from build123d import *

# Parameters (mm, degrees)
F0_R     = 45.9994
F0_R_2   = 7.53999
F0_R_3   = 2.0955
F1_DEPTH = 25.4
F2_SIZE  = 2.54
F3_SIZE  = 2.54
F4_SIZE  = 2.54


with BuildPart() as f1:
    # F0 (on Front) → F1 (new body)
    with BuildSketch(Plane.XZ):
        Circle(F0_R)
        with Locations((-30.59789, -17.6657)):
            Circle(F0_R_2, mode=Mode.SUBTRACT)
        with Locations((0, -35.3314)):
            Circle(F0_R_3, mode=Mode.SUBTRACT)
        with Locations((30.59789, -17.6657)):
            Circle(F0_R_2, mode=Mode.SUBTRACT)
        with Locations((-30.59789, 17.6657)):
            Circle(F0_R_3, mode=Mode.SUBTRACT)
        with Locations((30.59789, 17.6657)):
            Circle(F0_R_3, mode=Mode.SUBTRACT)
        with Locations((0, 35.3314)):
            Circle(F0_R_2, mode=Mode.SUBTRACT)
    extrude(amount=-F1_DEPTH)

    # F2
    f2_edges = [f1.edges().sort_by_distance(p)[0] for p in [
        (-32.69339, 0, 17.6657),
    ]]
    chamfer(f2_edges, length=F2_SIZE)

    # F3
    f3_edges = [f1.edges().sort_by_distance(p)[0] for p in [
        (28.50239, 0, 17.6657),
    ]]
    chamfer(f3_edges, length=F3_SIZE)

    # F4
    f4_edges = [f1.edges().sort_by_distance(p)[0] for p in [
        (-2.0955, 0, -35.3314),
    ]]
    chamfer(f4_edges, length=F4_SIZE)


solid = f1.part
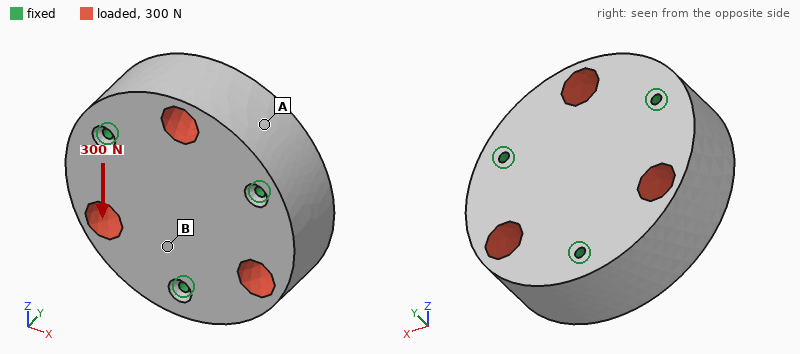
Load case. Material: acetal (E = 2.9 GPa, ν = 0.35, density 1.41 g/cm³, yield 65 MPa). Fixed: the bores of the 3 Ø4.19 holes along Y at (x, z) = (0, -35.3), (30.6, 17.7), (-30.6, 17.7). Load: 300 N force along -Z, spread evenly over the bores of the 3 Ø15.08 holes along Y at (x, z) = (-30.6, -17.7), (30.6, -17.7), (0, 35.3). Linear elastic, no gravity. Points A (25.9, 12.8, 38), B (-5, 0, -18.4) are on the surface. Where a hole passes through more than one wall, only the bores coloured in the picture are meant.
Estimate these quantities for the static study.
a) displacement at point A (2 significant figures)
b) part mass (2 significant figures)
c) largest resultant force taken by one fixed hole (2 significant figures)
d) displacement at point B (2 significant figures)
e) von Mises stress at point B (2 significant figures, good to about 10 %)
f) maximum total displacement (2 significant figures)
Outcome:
0.88 µm
220 g
110 N
0.91 µm
0.11 MPa
3.4 µm
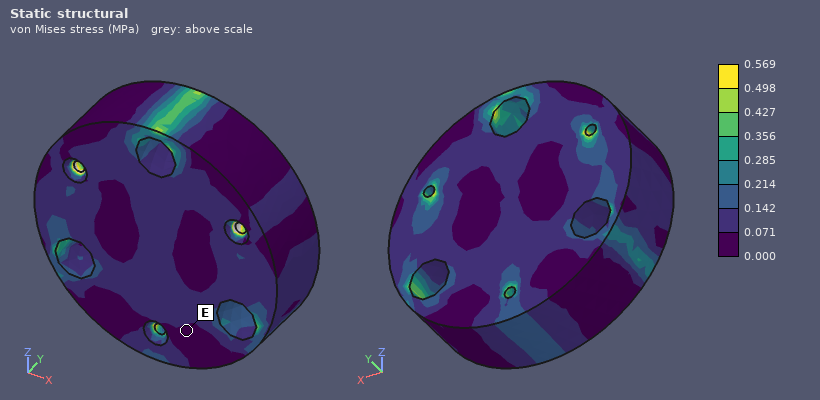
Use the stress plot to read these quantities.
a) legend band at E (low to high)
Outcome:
0.000 to 0.071 MPa
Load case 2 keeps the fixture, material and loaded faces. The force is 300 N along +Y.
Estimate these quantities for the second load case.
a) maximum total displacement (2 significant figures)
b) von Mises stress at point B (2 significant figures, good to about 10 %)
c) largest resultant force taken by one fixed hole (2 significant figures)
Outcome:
8.2 µm
0.22 MPa
100 N
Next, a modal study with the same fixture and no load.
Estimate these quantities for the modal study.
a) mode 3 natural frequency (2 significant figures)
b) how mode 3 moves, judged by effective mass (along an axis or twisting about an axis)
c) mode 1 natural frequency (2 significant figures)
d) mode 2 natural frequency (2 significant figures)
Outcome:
3800 Hz
along Y
3600 Hz
3600 Hz
